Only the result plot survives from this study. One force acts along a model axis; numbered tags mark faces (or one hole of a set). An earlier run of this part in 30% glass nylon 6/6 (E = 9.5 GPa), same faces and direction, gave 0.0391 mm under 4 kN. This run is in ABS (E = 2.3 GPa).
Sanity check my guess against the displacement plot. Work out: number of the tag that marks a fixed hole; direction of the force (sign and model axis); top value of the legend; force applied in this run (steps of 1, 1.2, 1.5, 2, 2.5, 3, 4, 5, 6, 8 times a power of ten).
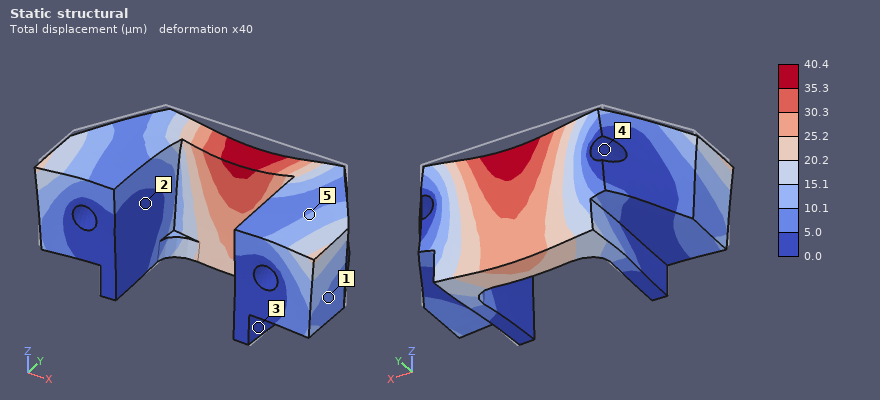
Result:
4
-Z
40.4 µm
1 kN
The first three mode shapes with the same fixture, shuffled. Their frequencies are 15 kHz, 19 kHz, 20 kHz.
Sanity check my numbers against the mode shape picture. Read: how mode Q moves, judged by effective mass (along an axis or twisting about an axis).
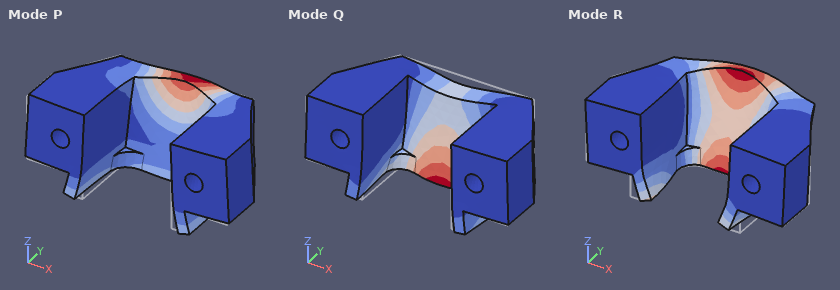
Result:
along Y
